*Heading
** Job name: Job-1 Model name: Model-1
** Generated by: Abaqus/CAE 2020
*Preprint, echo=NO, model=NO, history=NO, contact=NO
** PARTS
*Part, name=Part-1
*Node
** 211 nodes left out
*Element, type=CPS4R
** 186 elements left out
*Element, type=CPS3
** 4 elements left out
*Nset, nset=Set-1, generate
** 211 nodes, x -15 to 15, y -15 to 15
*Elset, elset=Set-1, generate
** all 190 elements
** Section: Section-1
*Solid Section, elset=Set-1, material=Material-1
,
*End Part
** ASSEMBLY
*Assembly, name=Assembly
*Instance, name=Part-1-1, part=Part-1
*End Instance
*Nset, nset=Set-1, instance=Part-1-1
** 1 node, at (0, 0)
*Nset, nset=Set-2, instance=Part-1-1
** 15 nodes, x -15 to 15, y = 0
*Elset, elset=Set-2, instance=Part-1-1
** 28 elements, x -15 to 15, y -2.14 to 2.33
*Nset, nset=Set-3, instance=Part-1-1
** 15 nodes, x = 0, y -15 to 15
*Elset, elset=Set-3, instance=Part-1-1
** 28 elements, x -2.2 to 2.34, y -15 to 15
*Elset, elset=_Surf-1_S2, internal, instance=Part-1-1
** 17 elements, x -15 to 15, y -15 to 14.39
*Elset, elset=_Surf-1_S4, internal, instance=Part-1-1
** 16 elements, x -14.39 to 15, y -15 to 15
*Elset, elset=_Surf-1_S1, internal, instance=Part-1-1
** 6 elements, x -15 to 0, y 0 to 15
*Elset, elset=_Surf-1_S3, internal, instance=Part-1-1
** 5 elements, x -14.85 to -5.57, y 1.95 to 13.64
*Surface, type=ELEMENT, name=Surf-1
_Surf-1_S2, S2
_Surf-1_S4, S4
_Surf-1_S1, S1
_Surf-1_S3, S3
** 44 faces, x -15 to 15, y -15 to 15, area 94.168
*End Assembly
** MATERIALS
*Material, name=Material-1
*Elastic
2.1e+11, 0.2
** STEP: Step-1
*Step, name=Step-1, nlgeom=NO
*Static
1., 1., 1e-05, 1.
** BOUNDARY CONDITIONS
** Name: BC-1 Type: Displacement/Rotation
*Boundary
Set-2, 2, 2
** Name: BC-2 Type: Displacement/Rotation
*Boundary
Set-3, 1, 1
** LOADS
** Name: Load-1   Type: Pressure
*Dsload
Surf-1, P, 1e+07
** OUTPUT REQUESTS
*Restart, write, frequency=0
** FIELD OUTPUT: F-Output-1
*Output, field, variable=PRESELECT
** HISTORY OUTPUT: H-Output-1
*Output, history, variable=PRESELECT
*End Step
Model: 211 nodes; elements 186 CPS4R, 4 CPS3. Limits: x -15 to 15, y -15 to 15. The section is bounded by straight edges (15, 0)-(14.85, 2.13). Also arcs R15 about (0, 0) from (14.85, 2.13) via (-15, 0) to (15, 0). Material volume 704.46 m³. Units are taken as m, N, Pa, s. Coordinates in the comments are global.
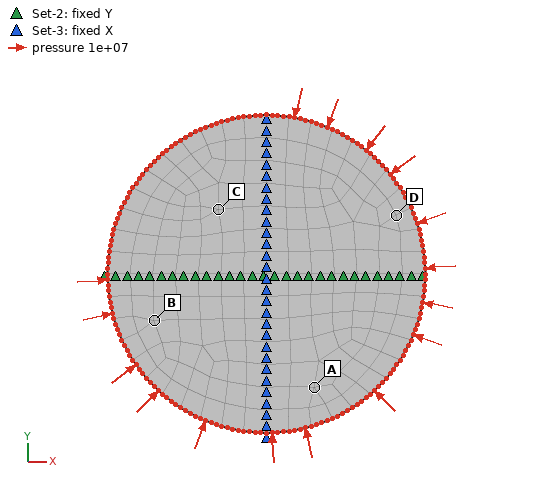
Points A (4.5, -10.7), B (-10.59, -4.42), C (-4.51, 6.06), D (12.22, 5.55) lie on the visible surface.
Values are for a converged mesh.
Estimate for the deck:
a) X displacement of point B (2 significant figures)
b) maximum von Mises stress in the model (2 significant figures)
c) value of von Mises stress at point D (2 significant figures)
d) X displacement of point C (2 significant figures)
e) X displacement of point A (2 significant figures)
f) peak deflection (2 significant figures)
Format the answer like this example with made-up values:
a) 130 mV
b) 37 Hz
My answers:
a) 4.0e-04 m
b) 1.0e+07 Pa
c) 1.0e+07 Pa
d) 1.7e-04 m
e) -1.7e-04 m
f) 5.7e-04 m
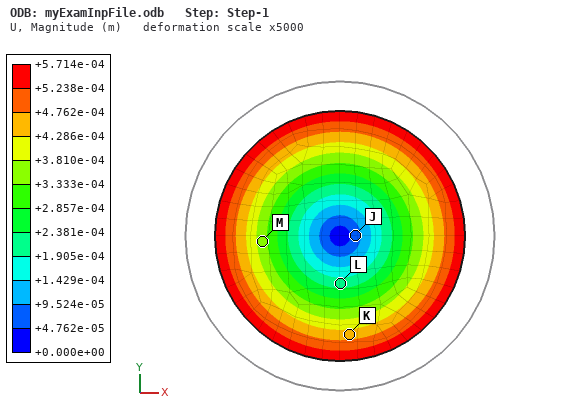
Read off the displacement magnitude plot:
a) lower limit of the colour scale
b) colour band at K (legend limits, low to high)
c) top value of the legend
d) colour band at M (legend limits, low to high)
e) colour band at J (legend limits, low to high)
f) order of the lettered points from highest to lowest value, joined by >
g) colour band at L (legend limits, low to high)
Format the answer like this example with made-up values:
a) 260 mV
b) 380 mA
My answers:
a) +0.000e+00 m
b) +4.286e-04 to +4.762e-04 m
c) +5.714e-04 m
d) +3.333e-04 to +3.810e-04 m
e) +4.762e-05 to +9.524e-05 m
f) K > M > L > J
g) +1.905e-04 to +2.381e-04 m
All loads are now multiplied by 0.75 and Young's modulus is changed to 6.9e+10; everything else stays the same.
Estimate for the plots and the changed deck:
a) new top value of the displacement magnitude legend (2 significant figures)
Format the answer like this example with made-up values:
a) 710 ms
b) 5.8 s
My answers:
a) 0.0013 m
